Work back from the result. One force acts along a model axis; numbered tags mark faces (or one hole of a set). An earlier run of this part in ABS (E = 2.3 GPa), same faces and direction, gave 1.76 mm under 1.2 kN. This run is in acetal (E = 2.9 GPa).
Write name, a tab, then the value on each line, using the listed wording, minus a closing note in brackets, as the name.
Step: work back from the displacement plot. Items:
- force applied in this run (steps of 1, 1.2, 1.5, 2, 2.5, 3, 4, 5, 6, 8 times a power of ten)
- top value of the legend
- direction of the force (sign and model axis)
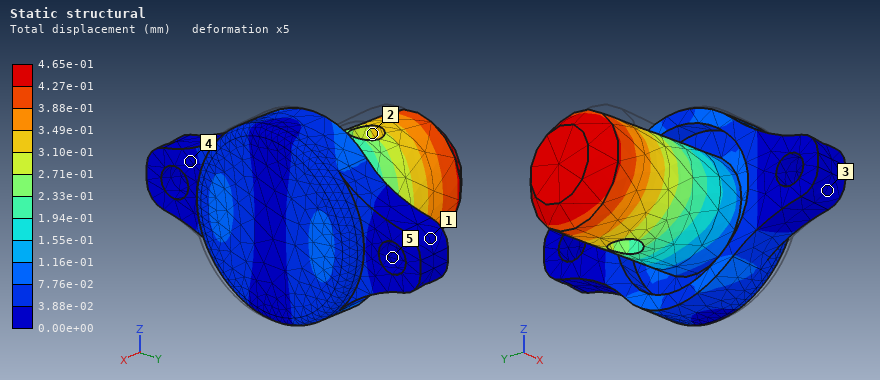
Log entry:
force applied in this run	400 N
top value of the legend	4.65e-01 mm
direction of the force	+Y
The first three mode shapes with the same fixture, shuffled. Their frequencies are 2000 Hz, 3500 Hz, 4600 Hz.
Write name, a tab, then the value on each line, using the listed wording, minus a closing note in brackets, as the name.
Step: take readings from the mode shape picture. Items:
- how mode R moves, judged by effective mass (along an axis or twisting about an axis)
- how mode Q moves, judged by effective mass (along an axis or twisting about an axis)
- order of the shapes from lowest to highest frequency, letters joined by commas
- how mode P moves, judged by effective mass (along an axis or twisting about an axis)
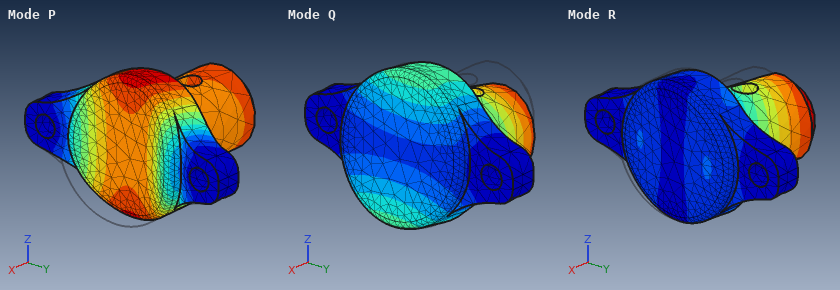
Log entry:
how mode R moves, judged by effective mass	along Y
how mode Q moves, judged by effective mass	along Z
order of the shapes from lowest to highest frequency, letters joined by commas	Q, R, P
how mode P moves, judged by effective mass	along X
